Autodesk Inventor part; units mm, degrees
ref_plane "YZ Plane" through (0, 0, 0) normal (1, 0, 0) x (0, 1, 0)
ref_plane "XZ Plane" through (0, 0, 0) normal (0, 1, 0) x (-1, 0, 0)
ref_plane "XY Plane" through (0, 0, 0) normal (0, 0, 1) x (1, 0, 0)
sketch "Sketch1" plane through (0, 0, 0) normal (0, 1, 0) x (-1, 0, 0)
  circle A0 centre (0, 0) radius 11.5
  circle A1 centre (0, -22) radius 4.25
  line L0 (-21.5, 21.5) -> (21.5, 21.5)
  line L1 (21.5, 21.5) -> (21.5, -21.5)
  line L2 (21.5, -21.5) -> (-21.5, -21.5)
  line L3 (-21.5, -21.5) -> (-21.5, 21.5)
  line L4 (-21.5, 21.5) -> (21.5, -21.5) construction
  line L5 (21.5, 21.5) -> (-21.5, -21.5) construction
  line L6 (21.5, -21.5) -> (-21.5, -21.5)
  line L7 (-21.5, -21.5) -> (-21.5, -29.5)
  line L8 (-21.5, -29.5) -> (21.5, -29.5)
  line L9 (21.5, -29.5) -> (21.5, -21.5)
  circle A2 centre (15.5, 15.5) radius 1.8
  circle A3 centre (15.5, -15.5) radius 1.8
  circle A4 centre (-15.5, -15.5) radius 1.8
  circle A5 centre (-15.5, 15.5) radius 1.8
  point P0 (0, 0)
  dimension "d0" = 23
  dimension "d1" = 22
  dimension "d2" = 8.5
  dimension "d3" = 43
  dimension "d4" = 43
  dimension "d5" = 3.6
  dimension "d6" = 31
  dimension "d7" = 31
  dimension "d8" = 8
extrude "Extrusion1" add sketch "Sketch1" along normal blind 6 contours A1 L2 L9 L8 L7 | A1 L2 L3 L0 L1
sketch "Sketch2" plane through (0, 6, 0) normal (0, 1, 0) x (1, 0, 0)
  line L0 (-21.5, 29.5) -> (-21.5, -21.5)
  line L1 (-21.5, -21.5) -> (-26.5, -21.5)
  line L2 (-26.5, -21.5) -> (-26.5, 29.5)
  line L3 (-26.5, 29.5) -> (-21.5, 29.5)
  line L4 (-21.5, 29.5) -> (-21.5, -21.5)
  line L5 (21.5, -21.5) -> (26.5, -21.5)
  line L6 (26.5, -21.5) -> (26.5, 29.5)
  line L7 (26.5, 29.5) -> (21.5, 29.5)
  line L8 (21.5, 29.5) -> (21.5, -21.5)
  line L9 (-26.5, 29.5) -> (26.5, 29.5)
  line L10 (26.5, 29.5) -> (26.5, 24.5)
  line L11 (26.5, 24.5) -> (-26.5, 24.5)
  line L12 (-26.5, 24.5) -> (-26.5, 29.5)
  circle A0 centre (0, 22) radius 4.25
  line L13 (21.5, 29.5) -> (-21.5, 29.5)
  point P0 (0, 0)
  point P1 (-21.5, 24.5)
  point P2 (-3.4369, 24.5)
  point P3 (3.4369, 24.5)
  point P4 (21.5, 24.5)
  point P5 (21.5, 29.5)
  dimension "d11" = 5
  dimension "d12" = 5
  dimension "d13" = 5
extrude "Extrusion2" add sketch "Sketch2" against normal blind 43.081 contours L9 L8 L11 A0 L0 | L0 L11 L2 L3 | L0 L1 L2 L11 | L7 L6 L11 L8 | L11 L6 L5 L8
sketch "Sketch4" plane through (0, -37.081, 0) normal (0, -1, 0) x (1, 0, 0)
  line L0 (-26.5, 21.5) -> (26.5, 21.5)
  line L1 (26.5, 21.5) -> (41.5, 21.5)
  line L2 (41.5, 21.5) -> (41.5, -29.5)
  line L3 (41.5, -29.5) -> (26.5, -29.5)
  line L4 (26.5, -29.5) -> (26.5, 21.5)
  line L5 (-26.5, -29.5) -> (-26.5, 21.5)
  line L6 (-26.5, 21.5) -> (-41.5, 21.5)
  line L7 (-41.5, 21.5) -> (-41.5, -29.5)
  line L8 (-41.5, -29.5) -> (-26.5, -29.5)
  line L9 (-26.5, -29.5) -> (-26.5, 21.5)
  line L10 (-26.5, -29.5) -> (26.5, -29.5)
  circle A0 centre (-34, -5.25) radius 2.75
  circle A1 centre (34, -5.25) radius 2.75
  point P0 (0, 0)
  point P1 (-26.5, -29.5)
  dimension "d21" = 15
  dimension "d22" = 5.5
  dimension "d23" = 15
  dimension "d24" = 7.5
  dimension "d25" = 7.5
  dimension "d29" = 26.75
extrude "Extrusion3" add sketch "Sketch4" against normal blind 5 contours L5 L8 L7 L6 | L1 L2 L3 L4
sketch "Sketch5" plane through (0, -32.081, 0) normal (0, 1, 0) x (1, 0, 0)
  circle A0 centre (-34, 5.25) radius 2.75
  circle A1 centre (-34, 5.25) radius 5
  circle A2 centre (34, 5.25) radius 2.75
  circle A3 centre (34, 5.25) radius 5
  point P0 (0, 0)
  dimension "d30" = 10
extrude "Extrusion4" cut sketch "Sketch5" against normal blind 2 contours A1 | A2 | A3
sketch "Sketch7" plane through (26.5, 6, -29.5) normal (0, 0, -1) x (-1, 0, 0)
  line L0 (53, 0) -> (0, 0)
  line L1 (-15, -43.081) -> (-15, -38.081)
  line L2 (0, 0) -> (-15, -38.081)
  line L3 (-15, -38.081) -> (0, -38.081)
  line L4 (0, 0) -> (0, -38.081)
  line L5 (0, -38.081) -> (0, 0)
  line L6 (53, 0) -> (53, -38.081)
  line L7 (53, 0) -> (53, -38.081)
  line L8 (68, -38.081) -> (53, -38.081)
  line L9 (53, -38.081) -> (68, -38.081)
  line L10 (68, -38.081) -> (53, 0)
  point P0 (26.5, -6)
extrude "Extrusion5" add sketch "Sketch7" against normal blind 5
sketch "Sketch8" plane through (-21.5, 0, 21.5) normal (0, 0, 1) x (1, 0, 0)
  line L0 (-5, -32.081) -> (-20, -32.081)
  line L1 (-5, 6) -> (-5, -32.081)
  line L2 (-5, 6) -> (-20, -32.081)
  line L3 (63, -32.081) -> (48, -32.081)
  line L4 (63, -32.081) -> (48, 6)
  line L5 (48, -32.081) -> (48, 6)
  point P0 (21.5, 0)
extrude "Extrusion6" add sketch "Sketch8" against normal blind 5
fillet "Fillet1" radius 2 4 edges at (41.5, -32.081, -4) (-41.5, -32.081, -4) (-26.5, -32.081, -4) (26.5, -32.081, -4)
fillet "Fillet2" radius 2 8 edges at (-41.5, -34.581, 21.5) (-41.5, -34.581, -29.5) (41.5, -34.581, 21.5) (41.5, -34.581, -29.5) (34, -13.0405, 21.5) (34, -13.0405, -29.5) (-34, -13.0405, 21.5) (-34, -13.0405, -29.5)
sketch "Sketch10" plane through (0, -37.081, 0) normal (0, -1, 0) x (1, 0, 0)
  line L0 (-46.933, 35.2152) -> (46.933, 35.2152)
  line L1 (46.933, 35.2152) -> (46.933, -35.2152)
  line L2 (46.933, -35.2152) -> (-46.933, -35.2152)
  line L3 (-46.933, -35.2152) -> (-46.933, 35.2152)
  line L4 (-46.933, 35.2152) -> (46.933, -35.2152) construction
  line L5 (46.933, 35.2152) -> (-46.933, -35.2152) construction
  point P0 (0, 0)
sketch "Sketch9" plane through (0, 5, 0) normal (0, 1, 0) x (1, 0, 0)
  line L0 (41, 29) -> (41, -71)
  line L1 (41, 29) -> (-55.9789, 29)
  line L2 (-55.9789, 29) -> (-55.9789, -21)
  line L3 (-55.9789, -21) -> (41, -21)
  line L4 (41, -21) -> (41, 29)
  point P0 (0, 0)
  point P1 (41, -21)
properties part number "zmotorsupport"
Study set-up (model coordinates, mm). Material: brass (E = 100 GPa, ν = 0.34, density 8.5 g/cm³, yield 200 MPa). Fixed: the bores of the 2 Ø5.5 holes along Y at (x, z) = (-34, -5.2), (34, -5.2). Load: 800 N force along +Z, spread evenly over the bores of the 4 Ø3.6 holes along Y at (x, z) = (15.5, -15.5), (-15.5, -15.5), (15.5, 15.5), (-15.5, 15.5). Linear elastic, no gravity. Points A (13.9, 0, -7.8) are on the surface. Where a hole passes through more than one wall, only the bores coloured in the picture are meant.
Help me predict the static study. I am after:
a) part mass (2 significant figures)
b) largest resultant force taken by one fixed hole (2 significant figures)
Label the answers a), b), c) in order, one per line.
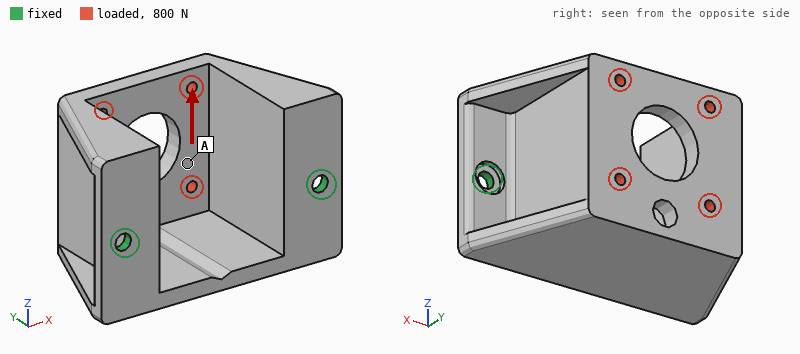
a) 450 g
b) 460 N
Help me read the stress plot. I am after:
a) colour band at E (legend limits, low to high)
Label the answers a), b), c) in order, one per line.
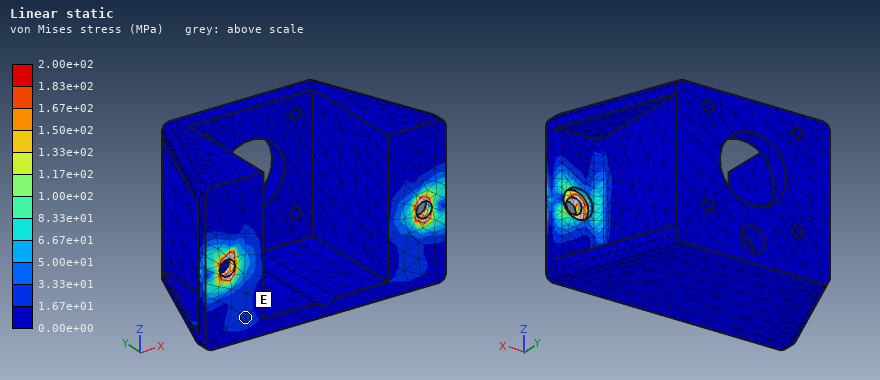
a) 1.67e+01 to 3.33e+01 MPa
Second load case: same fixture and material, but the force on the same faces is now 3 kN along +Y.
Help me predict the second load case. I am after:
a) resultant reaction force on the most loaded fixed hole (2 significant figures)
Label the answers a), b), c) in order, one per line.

a) 1.6 kN
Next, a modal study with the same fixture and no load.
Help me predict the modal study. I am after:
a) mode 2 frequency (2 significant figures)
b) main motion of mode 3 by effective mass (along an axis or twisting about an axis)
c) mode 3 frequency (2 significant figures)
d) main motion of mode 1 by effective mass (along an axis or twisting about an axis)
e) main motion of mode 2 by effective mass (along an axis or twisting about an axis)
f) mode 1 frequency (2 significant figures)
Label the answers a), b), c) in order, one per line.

a) 1600 Hz
b) along X
c) 3000 Hz
d) along Z
e) along X
f) 670 Hz
